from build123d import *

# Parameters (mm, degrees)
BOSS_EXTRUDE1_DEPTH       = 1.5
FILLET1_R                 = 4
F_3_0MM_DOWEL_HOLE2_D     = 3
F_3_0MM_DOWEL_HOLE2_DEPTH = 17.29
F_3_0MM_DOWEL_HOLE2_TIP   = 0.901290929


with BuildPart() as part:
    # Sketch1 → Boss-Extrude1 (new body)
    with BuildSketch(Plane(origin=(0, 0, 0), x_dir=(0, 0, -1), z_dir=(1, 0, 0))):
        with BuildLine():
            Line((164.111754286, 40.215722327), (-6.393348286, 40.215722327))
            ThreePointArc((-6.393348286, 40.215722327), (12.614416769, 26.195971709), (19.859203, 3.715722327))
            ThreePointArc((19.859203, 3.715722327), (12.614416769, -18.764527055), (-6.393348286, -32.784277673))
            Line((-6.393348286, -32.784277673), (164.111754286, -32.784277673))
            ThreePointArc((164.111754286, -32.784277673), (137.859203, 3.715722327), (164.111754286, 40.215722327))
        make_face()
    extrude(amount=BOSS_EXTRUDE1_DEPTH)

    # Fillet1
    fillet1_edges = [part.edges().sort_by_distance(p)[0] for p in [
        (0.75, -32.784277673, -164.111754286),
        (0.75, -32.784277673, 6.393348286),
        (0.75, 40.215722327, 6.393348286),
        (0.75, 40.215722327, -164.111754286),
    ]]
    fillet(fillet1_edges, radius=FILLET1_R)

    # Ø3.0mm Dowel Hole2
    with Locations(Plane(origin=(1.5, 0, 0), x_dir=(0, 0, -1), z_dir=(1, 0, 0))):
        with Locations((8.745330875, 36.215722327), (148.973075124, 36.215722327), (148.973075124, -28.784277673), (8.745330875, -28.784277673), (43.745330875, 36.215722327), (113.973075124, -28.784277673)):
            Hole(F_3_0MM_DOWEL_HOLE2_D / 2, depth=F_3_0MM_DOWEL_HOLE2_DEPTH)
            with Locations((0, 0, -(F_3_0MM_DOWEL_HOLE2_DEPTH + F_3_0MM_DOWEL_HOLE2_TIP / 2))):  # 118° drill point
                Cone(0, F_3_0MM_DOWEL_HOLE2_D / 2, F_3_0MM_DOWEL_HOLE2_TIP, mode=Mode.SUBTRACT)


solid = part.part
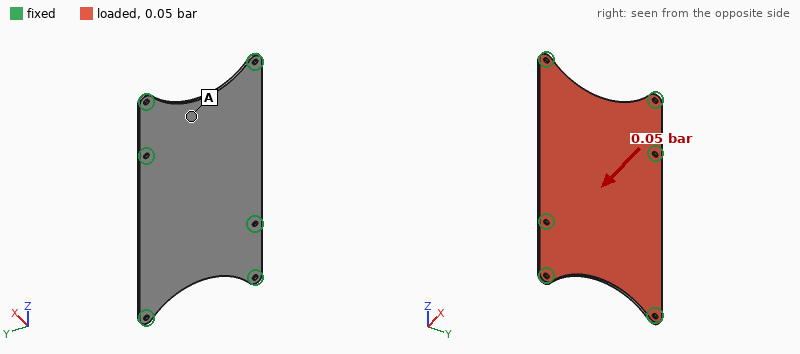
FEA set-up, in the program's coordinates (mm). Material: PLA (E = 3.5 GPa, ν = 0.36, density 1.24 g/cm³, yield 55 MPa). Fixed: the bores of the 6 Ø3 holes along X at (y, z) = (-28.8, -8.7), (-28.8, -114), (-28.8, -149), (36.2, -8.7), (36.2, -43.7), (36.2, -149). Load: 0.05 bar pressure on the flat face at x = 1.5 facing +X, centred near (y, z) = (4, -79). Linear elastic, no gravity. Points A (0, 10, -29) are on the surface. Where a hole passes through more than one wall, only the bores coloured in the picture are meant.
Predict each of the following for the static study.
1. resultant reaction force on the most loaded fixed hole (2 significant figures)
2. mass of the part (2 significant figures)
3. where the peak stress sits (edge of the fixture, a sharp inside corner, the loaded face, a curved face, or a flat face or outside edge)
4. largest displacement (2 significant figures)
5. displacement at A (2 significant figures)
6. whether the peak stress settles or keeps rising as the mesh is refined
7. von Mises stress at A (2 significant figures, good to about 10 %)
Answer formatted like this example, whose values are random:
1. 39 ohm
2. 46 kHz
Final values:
1. 17 N
2. 18 g
3. edge of the fixture
4. 1.8 mm
5. 0.52 mm
6. keeps rising
7. 3.4 MPa
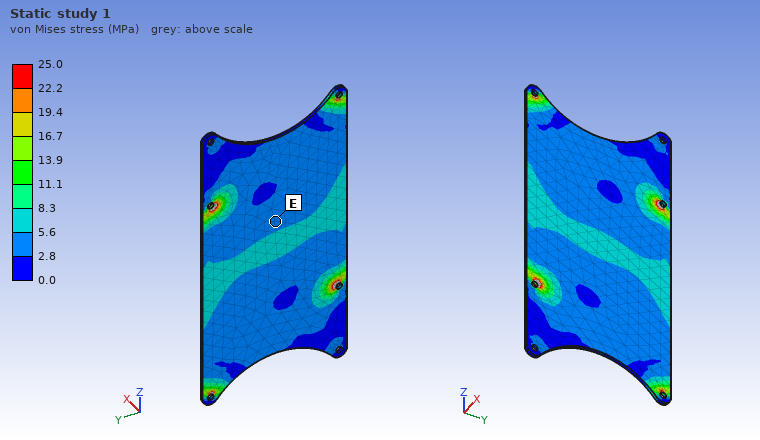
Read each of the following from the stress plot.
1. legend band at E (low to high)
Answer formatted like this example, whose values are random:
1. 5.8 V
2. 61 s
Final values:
1. 2.8 to 5.6 MPa
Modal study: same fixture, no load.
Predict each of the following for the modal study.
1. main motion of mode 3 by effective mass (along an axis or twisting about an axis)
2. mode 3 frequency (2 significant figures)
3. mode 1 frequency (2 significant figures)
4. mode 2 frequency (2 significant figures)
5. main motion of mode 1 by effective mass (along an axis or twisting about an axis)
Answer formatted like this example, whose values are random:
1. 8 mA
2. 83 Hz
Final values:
1. twisting about Y
2. 560 Hz
3. 230 Hz
4. 270 Hz
5. along X
